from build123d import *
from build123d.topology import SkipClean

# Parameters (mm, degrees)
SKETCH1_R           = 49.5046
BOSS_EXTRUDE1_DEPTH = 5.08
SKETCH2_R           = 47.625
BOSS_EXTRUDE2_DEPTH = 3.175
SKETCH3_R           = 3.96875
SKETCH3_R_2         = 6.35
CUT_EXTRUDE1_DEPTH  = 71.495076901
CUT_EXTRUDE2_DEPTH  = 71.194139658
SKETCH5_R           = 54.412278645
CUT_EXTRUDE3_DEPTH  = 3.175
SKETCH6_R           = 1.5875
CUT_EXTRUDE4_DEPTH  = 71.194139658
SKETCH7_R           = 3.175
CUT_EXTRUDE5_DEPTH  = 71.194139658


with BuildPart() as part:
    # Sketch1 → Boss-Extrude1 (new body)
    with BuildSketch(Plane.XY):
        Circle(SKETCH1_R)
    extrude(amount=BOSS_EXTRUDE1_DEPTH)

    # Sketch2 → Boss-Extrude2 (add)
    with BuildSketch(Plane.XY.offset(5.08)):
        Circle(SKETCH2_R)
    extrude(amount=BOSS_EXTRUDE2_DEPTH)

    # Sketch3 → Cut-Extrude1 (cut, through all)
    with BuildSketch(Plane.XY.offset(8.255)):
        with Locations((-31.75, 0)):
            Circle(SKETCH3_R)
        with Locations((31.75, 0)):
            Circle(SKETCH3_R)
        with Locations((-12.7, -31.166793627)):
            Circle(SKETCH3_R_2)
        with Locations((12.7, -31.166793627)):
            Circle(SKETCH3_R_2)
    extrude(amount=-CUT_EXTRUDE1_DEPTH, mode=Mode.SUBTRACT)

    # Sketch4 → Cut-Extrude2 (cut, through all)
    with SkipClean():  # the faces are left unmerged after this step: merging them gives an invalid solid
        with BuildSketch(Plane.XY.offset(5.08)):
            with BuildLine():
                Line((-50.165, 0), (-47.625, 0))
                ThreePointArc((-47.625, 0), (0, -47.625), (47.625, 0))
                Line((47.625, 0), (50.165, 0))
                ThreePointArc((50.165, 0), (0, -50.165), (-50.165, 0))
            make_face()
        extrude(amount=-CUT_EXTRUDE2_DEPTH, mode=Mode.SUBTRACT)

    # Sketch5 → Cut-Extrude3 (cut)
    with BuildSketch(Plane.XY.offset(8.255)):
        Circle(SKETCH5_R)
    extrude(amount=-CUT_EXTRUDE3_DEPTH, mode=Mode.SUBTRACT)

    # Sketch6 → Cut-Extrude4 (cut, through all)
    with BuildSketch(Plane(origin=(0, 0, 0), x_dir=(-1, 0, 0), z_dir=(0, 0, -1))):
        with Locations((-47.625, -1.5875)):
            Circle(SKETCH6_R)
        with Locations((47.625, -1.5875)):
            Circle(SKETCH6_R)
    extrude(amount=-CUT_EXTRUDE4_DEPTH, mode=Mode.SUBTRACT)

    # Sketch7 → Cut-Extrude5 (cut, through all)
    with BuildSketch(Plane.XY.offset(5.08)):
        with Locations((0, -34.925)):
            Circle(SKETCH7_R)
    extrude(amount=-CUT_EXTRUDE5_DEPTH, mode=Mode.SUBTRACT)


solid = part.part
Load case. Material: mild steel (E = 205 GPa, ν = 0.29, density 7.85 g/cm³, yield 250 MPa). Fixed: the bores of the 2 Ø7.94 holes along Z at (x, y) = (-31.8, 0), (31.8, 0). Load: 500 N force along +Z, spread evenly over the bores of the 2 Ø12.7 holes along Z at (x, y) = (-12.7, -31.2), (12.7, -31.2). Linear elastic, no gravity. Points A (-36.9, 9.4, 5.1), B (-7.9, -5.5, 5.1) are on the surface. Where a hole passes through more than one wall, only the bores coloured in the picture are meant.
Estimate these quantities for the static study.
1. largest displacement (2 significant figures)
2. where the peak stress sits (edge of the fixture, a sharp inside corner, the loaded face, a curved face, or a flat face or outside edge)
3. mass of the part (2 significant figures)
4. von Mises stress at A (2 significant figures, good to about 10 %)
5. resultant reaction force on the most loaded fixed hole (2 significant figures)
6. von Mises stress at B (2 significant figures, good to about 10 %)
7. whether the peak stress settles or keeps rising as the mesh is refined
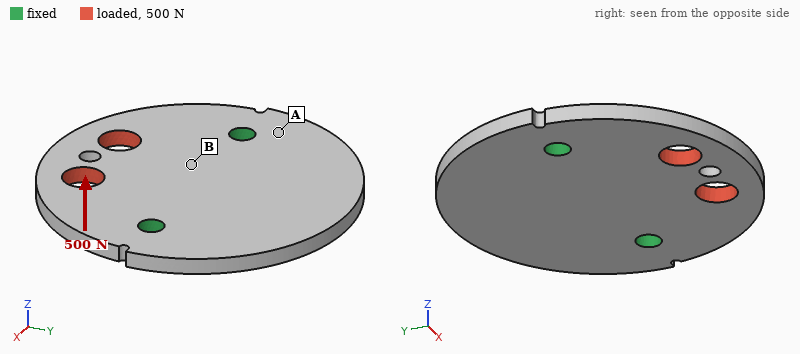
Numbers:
65 µm
edge of the fixture
280 g
8.1 MPa
250 N
22 MPa
keeps rising
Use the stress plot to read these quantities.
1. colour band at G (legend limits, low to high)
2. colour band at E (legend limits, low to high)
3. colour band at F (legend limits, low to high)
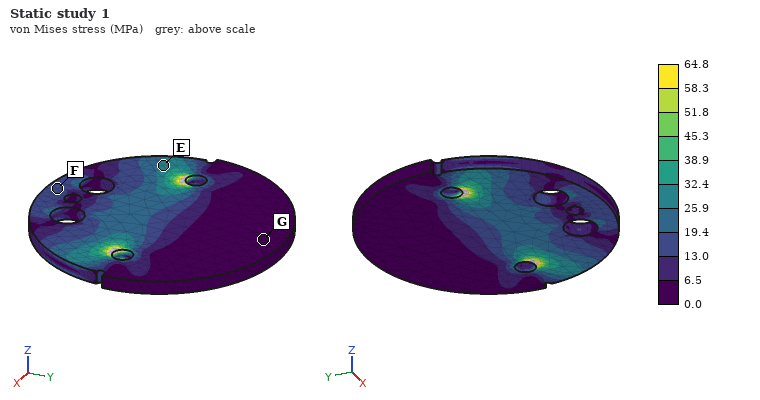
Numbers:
0.0 to 6.5 MPa
25.9 to 32.4 MPa
13.0 to 19.4 MPa
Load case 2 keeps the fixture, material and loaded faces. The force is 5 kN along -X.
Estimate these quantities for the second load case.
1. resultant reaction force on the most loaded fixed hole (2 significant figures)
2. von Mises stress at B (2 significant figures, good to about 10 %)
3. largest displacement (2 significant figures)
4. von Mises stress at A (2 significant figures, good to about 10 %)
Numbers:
3.4 kN
17 MPa
9.6 µm
10 MPa
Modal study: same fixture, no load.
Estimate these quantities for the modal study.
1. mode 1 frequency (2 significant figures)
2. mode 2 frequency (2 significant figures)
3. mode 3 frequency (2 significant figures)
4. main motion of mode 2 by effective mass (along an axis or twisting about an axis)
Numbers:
2000 Hz
2500 Hz
4700 Hz
along Z
